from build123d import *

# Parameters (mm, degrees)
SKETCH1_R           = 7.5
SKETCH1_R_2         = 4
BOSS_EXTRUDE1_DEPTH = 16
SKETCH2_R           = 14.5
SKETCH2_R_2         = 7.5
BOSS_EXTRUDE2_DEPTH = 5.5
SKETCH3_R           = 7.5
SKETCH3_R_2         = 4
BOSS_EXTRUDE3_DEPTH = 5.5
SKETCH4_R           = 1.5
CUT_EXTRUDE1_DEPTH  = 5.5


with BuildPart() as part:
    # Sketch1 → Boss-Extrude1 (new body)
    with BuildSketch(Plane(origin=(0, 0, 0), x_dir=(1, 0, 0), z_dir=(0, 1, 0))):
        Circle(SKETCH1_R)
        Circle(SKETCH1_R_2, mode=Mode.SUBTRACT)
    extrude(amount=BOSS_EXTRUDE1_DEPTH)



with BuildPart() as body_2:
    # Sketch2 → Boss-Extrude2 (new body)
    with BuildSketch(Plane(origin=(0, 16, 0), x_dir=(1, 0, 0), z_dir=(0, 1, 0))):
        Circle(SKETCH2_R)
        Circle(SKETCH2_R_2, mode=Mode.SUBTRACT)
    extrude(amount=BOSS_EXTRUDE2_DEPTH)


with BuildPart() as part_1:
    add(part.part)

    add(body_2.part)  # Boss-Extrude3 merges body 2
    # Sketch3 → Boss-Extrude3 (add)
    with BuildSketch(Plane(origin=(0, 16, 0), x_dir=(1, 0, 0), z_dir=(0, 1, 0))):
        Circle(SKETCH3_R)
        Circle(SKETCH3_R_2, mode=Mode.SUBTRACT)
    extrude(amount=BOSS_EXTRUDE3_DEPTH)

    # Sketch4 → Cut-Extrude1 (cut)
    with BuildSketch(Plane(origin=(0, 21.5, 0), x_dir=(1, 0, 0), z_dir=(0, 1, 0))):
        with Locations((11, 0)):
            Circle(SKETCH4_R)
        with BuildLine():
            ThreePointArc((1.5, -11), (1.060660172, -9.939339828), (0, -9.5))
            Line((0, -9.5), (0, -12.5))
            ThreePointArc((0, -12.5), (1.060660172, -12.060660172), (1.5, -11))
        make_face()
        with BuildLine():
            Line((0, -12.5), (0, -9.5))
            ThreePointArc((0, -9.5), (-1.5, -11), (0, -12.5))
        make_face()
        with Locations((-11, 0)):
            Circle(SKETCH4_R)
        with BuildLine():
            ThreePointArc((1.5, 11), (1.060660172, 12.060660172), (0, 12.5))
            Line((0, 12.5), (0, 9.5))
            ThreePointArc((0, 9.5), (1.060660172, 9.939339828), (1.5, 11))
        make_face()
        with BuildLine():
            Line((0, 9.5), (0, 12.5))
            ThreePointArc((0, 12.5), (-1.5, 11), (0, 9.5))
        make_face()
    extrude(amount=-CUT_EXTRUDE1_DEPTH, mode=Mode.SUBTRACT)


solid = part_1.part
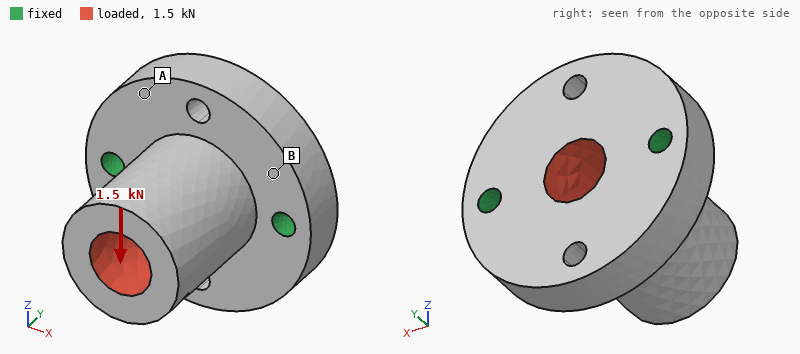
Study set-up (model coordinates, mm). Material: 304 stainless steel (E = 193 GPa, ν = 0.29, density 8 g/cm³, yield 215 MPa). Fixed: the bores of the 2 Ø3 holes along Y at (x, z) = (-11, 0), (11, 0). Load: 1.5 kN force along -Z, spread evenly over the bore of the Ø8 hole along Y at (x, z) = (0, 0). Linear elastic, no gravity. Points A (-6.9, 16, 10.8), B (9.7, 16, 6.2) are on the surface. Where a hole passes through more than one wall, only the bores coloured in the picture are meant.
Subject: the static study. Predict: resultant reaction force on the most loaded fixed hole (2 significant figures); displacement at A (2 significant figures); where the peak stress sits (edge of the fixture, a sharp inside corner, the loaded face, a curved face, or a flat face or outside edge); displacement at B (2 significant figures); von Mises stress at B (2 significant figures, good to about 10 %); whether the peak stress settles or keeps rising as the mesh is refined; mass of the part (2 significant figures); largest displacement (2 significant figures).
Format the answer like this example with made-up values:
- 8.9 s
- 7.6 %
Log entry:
- 750 N
- 6.6 µm
- edge of the fixture
- 3.2 µm
- 31 MPa
- keeps rising
- 42 g
- 18 µm
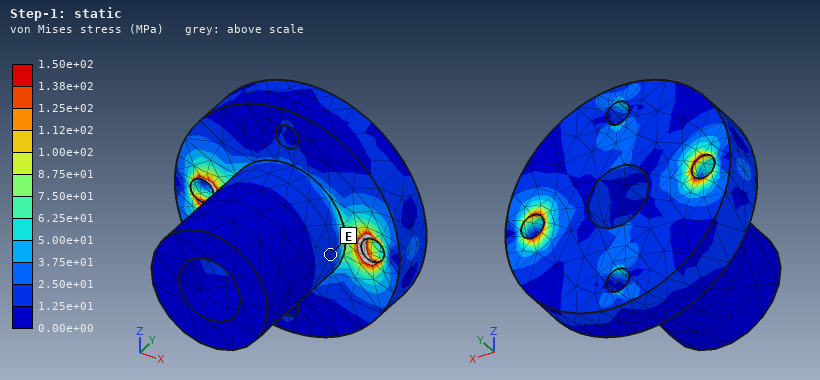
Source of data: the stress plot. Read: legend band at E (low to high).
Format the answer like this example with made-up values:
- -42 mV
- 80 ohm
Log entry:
- 1.25e+01 to 2.50e+01 MPa
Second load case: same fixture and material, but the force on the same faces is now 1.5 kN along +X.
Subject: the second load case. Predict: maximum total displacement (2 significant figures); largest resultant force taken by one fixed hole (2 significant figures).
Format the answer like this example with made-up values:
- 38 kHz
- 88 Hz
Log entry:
- 5.8 µm
- 980 N
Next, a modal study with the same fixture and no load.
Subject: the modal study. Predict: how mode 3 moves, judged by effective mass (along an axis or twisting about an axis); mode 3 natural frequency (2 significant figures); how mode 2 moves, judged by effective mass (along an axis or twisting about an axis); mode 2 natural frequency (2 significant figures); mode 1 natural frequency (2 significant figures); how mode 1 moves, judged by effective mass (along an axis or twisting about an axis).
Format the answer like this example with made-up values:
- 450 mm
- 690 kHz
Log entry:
- along Y
- 23 kHz
- along X
- 20 kHz
- 10 kHz
- along Z
